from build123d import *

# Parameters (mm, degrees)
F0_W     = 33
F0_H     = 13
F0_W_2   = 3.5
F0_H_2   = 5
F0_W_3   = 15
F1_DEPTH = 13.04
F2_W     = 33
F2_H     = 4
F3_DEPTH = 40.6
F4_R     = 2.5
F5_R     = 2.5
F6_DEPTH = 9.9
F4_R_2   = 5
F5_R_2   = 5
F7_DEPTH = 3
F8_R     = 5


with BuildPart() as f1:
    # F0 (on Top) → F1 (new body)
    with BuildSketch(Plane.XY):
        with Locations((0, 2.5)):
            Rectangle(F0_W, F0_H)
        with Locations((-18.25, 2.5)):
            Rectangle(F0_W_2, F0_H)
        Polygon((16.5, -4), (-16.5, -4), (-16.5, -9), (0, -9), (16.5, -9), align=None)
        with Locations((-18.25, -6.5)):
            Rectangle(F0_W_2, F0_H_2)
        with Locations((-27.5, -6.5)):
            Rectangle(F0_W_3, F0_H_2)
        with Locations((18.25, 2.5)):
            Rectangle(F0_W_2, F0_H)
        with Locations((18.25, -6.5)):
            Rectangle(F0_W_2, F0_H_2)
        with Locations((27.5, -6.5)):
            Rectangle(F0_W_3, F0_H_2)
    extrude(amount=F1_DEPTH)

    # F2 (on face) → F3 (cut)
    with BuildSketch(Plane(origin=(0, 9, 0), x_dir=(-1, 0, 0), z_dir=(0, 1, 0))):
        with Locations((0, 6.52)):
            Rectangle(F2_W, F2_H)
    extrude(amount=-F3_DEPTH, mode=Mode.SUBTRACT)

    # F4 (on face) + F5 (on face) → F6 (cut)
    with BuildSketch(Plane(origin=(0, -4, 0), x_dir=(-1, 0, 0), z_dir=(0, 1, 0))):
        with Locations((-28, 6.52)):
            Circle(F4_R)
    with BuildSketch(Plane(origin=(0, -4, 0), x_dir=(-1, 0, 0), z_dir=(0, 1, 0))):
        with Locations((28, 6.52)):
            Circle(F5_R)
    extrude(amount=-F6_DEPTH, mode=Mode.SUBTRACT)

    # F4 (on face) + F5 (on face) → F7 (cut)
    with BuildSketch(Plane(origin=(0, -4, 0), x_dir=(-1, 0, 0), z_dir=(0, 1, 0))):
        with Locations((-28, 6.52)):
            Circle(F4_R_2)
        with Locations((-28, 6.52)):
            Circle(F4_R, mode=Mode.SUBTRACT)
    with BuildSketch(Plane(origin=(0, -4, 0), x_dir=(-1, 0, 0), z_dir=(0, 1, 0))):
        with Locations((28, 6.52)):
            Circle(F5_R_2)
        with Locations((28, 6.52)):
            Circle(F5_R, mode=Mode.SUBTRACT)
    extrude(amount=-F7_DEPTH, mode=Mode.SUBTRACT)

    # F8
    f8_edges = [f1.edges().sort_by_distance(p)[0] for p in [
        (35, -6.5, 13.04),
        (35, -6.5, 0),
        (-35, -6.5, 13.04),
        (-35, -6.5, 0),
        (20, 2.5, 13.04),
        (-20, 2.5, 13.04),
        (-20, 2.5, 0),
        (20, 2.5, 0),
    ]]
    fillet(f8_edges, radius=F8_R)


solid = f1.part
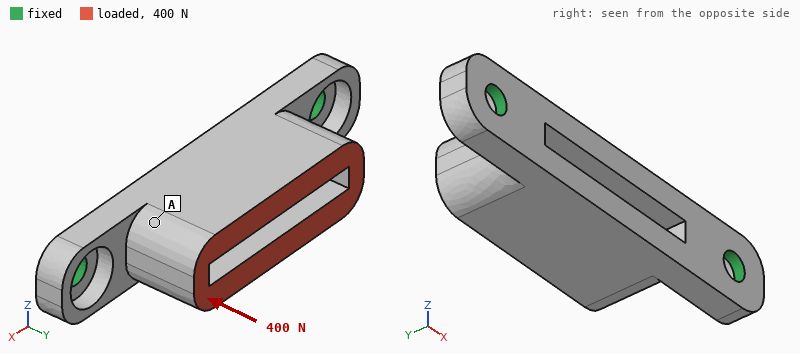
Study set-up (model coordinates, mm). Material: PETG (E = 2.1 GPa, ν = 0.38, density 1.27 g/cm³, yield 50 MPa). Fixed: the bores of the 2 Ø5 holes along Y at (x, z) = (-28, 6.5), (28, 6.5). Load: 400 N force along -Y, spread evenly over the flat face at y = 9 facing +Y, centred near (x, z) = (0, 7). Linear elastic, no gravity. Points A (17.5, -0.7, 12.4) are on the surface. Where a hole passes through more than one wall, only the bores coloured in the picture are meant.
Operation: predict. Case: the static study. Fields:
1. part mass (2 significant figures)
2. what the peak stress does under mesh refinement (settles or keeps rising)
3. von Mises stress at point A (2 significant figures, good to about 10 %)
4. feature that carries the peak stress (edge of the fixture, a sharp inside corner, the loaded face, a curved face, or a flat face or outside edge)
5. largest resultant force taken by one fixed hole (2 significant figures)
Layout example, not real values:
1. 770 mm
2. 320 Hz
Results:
1. 10 g
2. keeps rising
3. 4.2 MPa
4. edge of the fixture
5. 290 N
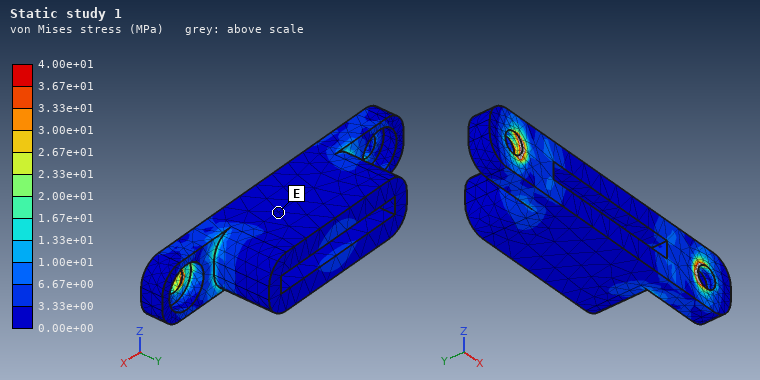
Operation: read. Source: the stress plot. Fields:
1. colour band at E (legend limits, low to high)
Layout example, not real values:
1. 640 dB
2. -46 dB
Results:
1. 0.00e+00 to 3.33e+00 MPa
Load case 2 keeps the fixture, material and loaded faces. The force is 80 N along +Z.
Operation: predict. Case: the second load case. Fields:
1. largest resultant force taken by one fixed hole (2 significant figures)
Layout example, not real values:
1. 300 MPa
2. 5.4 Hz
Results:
1. 40 N
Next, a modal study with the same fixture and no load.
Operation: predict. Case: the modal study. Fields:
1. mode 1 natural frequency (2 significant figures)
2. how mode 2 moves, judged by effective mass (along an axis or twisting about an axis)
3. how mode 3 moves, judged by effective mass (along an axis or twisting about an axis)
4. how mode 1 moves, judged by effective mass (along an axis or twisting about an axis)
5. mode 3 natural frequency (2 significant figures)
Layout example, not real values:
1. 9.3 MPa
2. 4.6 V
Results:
1. 960 Hz
2. along Y
3. twisting about Y
4. along Z
5. 3200 Hz
